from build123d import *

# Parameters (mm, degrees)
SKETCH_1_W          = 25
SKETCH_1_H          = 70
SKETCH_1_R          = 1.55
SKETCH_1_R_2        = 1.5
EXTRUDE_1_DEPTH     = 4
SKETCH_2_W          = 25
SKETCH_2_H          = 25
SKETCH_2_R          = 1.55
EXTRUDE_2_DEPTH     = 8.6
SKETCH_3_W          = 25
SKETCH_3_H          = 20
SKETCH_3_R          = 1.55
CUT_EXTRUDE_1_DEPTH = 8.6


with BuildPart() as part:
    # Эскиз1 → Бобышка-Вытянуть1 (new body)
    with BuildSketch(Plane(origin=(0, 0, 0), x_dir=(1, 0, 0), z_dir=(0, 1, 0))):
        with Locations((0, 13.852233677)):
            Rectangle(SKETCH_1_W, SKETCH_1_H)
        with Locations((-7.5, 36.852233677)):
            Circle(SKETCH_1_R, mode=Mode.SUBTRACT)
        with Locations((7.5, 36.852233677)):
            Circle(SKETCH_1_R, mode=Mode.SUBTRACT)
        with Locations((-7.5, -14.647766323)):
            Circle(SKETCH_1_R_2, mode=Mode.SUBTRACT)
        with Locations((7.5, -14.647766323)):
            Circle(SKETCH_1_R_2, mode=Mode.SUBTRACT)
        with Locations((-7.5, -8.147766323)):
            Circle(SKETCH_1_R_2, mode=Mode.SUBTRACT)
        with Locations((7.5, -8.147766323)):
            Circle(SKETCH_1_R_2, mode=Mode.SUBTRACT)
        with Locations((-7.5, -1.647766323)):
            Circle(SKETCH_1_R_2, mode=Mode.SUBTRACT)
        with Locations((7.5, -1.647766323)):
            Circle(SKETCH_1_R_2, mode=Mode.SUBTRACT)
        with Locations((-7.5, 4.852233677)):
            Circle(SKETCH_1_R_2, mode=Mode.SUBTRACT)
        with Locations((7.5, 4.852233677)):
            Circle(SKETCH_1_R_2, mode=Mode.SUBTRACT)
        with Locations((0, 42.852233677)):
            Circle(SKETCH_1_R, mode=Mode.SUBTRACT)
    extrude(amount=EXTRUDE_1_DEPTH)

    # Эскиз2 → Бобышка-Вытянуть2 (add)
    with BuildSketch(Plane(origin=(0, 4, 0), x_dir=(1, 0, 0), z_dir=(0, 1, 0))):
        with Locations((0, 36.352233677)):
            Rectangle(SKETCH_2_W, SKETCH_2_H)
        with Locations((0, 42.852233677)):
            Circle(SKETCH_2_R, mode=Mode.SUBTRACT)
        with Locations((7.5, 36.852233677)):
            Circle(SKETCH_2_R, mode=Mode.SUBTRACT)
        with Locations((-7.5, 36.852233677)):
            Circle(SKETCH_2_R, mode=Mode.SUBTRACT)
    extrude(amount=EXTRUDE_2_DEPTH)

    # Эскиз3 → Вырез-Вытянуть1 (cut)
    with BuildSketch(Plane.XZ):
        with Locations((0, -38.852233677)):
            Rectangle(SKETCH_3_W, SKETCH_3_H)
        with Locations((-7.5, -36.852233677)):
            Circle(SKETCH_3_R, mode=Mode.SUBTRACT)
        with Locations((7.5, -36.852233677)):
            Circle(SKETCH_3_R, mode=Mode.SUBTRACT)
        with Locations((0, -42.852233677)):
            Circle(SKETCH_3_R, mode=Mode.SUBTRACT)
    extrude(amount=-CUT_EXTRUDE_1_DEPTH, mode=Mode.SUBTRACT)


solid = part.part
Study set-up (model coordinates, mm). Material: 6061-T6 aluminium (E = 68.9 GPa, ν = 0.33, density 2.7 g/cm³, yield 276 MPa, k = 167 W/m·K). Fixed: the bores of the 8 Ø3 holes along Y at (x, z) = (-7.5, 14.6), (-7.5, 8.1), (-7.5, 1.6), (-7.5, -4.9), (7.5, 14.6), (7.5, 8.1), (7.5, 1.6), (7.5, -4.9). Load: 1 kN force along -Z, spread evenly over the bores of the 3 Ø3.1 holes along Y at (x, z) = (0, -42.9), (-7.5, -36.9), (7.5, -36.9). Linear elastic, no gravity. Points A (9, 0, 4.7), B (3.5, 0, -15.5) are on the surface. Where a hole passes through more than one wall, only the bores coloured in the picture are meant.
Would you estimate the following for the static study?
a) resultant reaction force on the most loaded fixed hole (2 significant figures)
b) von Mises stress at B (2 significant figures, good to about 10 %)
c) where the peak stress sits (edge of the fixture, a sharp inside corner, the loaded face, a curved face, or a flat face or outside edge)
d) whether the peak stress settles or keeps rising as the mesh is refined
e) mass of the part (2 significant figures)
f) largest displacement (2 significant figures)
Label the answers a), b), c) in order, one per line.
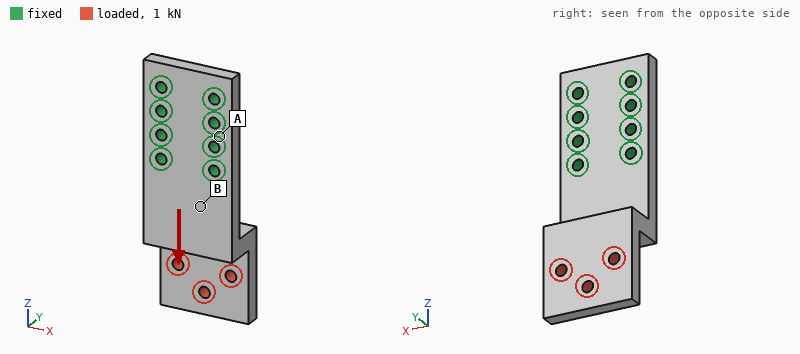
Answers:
a) 430 N
b) 110 MPa
c) edge of the fixture
d) keeps rising
e) 21 g
f) 0.69 mm
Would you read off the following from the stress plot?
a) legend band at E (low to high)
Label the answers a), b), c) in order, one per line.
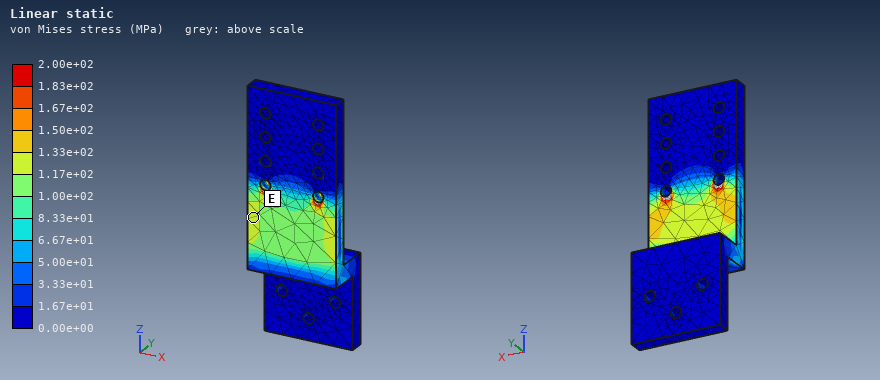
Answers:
a) 1.17e+02 to 1.33e+02 MPa
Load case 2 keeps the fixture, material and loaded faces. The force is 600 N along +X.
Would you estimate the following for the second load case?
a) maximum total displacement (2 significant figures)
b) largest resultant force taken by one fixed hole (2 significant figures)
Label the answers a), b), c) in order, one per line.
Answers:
a) 0.11 mm
b) 1.1 kN
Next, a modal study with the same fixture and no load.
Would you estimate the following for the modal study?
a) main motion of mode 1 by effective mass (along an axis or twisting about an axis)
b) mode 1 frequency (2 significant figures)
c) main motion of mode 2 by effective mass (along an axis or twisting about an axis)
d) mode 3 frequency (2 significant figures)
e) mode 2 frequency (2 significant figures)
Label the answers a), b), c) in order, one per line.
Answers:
a) along Y
b) 1600 Hz
c) along X
d) 7300 Hz
e) 4800 Hz
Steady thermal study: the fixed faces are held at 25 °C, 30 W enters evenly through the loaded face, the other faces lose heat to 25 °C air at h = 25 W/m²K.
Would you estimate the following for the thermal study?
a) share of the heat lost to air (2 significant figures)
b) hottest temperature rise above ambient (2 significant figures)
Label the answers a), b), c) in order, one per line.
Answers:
a) 9.9 %
b) 66 K
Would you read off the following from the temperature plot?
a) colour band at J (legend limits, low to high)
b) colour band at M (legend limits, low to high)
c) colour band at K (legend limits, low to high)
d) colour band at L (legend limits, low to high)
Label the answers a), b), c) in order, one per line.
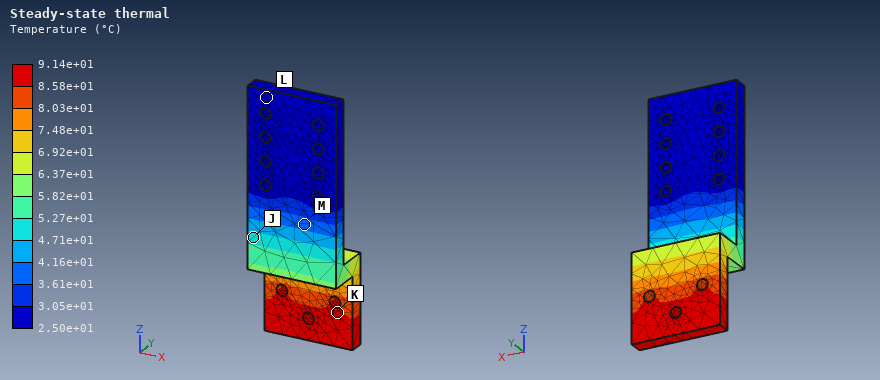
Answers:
a) 4.71e+01 to 5.27e+01 °C
b) 3.61e+01 to 4.16e+01 °C
c) 8.58e+01 to 9.14e+01 °C
d) 2.50e+01 to 3.05e+01 °C
